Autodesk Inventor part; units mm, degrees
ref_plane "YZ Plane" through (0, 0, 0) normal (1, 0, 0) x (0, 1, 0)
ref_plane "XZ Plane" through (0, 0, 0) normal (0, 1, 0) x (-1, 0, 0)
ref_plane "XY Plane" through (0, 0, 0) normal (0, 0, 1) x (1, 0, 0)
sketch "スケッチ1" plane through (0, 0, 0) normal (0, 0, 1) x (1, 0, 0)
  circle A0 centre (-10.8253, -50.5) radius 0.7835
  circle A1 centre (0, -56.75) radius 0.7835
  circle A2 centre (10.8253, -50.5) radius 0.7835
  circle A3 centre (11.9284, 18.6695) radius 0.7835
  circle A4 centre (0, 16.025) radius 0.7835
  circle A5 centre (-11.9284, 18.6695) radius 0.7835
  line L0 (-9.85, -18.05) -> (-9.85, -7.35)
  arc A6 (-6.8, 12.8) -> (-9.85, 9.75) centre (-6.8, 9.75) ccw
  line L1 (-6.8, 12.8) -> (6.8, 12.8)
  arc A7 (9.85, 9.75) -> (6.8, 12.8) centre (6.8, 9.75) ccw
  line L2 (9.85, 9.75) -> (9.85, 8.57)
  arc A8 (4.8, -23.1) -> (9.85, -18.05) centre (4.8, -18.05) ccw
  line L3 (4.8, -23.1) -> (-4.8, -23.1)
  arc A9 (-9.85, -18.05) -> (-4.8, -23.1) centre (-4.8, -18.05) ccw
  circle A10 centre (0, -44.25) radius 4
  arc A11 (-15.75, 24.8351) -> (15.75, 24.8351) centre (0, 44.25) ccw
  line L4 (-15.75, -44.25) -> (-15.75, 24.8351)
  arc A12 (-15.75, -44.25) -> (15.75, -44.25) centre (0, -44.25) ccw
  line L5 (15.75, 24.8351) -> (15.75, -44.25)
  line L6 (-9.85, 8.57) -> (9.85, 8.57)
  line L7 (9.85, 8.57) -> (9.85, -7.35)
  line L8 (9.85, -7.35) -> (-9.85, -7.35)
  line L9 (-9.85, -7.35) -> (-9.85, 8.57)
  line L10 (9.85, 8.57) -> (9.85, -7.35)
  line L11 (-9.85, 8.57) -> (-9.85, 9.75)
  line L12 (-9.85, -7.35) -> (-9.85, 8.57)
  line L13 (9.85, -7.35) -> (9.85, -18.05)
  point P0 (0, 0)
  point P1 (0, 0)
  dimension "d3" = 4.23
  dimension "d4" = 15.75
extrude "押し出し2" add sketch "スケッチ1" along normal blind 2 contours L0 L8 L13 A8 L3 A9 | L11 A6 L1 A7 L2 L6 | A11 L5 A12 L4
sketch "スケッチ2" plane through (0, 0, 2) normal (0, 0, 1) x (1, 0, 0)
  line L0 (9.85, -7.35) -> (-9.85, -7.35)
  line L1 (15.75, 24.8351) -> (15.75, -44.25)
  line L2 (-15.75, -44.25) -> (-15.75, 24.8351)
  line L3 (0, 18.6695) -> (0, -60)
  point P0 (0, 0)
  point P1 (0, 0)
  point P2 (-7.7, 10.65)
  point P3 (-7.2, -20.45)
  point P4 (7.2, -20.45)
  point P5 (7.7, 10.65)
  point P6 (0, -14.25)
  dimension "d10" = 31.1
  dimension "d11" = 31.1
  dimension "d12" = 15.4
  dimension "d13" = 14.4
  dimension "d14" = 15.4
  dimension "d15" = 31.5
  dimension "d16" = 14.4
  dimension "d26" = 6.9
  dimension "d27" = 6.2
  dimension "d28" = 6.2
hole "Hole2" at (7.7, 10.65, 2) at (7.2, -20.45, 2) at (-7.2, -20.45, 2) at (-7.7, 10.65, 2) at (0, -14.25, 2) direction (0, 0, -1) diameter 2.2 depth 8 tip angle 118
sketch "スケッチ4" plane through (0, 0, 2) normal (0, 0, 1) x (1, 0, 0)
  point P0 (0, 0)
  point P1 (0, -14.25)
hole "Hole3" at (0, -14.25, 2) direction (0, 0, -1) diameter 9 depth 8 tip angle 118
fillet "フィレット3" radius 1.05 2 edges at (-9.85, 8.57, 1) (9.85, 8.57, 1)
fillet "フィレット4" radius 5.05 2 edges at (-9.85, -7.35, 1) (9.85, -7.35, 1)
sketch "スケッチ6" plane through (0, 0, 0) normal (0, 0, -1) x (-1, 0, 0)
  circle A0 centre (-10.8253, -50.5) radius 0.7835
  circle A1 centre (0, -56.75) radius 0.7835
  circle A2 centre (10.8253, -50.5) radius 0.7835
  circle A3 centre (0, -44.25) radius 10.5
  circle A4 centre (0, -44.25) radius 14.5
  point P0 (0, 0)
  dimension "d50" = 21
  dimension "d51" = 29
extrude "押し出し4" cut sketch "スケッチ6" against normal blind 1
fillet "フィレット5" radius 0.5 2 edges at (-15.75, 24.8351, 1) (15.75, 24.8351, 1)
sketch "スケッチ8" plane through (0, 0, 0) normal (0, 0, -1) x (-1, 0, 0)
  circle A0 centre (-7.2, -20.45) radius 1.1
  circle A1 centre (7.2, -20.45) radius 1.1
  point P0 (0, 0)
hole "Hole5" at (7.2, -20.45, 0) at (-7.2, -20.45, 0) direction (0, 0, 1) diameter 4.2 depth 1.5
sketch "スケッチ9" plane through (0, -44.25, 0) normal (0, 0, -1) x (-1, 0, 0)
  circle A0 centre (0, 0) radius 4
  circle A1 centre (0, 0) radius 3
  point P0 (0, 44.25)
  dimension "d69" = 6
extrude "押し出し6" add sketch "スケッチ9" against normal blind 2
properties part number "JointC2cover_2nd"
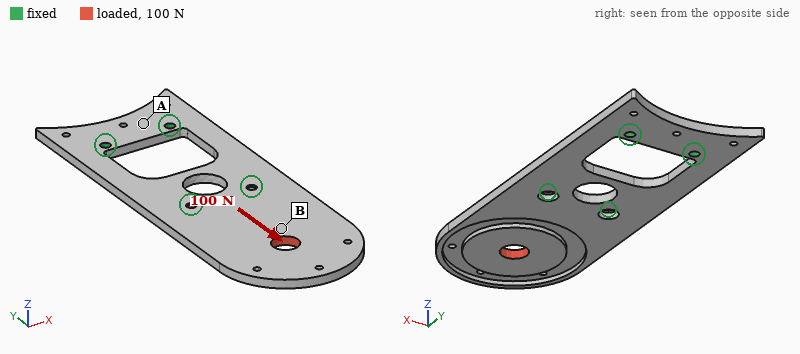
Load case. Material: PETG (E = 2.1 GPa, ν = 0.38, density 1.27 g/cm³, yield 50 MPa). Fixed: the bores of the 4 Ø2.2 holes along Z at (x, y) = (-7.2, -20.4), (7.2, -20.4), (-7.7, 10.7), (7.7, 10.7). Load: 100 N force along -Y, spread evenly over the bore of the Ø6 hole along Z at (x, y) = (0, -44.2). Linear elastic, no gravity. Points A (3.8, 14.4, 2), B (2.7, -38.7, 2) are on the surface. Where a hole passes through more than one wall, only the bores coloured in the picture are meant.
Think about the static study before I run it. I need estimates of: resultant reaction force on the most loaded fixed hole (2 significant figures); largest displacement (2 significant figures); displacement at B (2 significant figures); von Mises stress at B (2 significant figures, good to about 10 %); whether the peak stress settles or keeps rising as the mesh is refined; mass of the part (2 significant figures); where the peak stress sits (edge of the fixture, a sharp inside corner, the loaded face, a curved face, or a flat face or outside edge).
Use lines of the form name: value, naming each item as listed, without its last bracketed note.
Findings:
resultant reaction force on the most loaded fixed hole: 39 N
largest displacement: 0.96 mm
displacement at B: 0.31 mm
von Mises stress at B: 2.4 MPa
whether the peak stress settles or keeps rising as the mesh is refined: keeps rising
mass of the part: 4.7 g
where the peak stress sits: edge of the fixture
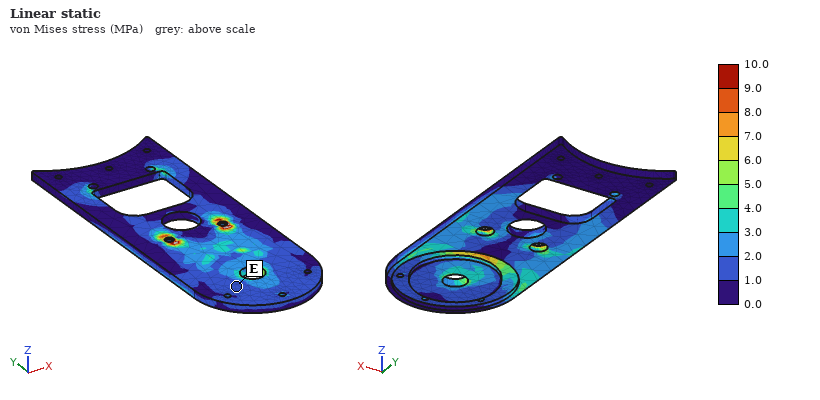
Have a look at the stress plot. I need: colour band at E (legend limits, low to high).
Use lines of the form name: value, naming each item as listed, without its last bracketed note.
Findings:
colour band at E: 1.0 to 2.0 MPa
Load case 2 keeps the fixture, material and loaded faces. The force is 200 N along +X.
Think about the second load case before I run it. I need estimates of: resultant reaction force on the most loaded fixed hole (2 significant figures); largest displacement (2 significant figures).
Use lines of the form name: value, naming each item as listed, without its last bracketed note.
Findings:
resultant reaction force on the most loaded fixed hole: 210 N
largest displacement: 0.72 mm
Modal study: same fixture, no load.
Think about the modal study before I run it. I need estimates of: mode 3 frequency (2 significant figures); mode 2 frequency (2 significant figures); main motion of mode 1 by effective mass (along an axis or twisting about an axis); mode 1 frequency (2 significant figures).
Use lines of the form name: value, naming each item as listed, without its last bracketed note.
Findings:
mode 3 frequency: 1300 Hz
mode 2 frequency: 790 Hz
main motion of mode 1 by effective mass: along Z
mode 1 frequency: 250 Hz
